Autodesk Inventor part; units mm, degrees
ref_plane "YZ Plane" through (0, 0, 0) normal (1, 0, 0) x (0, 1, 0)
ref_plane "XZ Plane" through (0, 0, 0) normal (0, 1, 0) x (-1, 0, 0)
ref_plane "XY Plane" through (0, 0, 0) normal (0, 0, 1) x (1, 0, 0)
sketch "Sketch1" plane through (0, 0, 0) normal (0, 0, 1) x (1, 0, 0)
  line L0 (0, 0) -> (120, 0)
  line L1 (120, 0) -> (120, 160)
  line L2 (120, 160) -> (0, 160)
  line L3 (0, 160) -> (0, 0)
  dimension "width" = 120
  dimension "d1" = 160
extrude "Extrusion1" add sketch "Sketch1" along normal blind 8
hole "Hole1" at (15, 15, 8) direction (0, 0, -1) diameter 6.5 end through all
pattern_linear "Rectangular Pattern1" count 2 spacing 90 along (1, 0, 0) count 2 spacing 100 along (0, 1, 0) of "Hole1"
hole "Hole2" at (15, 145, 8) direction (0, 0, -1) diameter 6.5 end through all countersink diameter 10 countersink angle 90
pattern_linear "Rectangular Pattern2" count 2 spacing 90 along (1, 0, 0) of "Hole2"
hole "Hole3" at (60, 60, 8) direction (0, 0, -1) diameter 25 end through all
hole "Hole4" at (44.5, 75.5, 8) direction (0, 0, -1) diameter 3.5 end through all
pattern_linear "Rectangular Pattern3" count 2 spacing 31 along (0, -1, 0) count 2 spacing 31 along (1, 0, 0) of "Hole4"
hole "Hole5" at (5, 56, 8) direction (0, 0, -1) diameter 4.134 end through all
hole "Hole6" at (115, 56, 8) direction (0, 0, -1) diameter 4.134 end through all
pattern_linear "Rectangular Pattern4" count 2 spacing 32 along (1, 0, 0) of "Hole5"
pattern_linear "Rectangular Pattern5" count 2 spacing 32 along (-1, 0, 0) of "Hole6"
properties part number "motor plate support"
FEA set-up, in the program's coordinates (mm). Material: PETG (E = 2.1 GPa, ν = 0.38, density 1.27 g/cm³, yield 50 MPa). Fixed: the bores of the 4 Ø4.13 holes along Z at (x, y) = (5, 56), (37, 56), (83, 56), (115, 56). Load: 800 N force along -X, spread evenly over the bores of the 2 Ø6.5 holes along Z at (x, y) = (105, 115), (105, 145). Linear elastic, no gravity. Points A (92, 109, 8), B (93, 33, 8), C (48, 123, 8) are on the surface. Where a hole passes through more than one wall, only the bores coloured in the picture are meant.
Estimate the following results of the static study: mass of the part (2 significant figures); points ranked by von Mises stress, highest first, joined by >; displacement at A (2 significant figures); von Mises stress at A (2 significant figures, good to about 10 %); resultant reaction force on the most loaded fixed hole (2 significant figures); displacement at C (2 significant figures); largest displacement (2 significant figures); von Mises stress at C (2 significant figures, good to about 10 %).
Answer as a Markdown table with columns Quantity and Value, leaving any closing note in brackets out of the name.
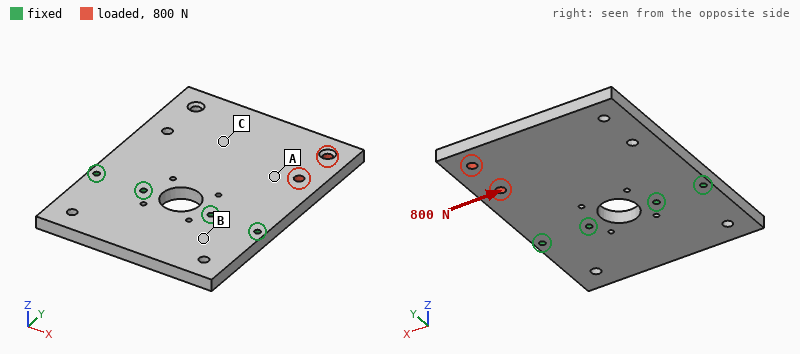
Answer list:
| Quantity | Value |
|---|---|
| mass of the part | 190 g |
| points ranked by von Mises stress, highest first, joined by > | A > C > B |
| displacement at A | 0.12 mm |
| von Mises stress at A | 2.2 MPa |
| resultant reaction force on the most loaded fixed hole | 530 N |
| displacement at C | 0.12 mm |
| largest displacement | 0.24 mm |
| von Mises stress at C | 1.2 MPa |
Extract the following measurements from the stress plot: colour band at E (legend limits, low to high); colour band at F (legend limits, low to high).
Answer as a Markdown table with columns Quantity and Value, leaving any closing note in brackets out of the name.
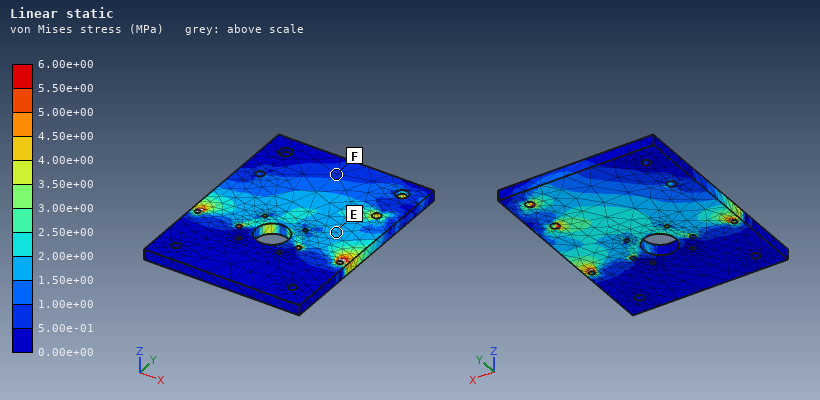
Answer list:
| Quantity | Value |
|---|---|
| colour band at E | 1.50e+00 to 2.00e+00 MPa |
| colour band at F | 5.00e-01 to 1.00e+00 MPa |
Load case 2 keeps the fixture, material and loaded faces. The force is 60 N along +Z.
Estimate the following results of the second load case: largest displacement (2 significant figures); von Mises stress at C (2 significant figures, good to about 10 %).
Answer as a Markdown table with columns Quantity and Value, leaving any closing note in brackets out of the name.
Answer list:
| Quantity | Value |
|---|---|
| largest displacement | 1.9 mm |
| von Mises stress at C | 1.1 MPa |
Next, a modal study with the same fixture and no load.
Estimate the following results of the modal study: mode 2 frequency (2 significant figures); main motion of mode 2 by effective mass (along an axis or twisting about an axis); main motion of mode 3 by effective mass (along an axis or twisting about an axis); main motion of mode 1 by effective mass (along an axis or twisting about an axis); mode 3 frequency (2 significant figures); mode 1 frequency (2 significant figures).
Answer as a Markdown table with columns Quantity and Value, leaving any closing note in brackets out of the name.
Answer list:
| Quantity | Value |
|---|---|
| mode 2 frequency | 330 Hz |
| main motion of mode 2 by effective mass | twisting about Y |
| main motion of mode 3 by effective mass | along Z |
| main motion of mode 1 by effective mass | along Z |
| mode 3 frequency | 460 Hz |
| mode 1 frequency | 140 Hz |
